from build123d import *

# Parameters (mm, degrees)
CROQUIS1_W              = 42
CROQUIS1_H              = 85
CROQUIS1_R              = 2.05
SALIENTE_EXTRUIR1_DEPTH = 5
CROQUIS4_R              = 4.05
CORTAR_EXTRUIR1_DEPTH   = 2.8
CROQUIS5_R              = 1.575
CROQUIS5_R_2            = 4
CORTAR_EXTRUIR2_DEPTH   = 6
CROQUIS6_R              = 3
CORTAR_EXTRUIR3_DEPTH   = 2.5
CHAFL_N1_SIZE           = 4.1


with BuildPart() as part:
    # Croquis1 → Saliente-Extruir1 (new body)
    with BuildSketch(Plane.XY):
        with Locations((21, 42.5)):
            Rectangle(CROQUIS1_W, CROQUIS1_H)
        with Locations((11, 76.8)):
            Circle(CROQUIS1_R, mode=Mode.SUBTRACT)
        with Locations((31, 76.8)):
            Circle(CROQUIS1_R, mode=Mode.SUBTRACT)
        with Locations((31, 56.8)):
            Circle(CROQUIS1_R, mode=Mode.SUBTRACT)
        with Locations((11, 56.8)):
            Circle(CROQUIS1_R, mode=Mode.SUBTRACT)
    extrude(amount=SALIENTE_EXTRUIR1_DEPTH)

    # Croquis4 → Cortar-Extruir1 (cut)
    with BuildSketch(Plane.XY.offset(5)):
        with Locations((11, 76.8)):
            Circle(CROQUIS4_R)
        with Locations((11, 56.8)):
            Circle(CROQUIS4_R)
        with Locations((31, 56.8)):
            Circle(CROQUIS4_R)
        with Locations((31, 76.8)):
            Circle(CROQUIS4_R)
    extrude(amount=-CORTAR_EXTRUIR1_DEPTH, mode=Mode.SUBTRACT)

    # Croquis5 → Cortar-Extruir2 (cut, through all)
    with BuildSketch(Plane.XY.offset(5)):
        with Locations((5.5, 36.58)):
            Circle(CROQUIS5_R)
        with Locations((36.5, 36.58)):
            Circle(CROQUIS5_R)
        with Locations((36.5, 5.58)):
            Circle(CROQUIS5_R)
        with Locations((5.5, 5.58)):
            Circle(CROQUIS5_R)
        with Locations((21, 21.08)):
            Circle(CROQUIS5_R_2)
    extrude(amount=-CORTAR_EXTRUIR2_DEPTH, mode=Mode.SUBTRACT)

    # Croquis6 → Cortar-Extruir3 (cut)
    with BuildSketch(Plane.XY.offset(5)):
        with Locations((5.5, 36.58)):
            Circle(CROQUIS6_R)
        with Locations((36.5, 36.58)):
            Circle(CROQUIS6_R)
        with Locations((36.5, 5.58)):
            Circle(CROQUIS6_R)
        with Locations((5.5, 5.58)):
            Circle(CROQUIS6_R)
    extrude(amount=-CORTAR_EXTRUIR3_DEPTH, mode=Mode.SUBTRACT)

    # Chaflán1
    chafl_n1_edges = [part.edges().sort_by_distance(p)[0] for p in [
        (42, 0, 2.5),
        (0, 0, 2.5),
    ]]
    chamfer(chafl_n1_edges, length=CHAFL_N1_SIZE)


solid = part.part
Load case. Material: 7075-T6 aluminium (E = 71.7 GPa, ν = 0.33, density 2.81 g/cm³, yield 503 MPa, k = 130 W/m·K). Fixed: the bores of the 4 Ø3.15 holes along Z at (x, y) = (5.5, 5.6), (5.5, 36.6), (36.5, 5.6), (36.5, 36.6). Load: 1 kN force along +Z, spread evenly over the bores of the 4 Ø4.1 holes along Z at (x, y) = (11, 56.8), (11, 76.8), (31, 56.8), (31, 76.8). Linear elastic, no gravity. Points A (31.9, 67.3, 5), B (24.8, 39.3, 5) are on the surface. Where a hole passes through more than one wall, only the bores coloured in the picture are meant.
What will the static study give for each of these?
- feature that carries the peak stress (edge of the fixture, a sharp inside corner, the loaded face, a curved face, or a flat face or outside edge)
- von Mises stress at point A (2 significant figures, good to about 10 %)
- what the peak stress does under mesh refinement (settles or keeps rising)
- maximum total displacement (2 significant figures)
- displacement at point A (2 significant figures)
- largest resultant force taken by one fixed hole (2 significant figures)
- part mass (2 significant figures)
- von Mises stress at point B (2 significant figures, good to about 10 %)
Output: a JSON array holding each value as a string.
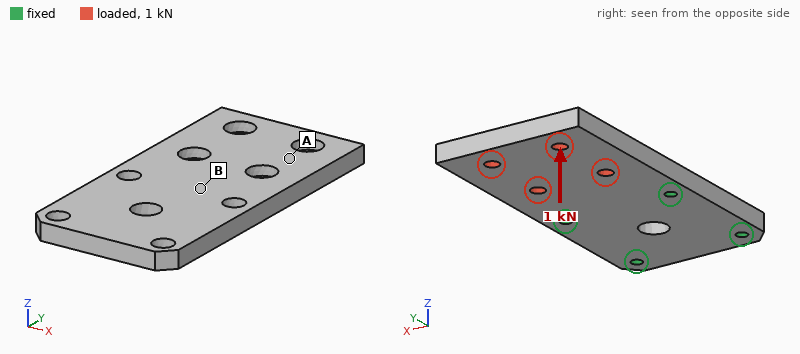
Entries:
["edge of the fixture", "33 MPa", "keeps rising", "0.91 mm", "0.50 mm", "1.4 kN", "46 g", "140 MPa"]
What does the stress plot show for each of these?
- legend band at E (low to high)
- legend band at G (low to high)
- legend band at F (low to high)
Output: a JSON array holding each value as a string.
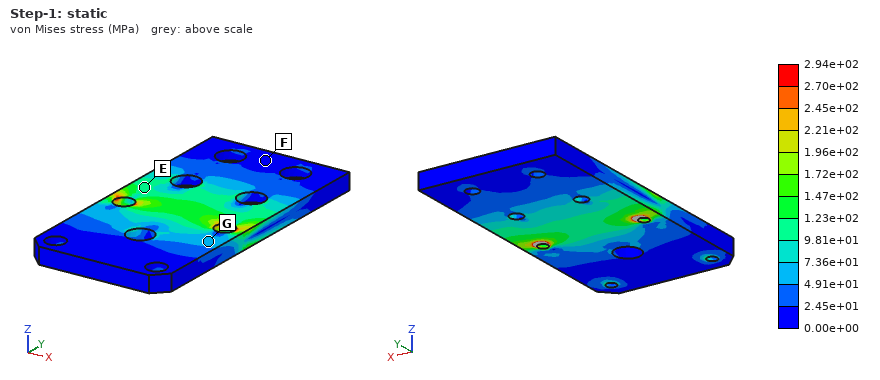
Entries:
["9.81e+01 to 1.23e+02 MPa", "4.91e+01 to 7.36e+01 MPa", "0.00e+00 to 2.45e+01 MPa"]
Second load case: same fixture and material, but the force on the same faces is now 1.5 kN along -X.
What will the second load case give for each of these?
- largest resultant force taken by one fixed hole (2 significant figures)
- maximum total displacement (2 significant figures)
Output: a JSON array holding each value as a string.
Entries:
["1.4 kN", "49 µm"]
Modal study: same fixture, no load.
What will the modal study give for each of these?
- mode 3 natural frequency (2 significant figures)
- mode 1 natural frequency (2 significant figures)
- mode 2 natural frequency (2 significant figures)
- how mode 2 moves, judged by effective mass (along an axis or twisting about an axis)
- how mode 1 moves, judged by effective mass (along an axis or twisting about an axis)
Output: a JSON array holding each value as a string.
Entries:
["8700 Hz", "1500 Hz", "4200 Hz", "twisting about Y", "along Z"]
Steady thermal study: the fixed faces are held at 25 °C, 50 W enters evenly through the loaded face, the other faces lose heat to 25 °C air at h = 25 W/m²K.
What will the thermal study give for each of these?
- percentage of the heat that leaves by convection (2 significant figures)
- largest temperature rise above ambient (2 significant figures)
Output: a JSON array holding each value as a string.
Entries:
["12 %", "71 K"]
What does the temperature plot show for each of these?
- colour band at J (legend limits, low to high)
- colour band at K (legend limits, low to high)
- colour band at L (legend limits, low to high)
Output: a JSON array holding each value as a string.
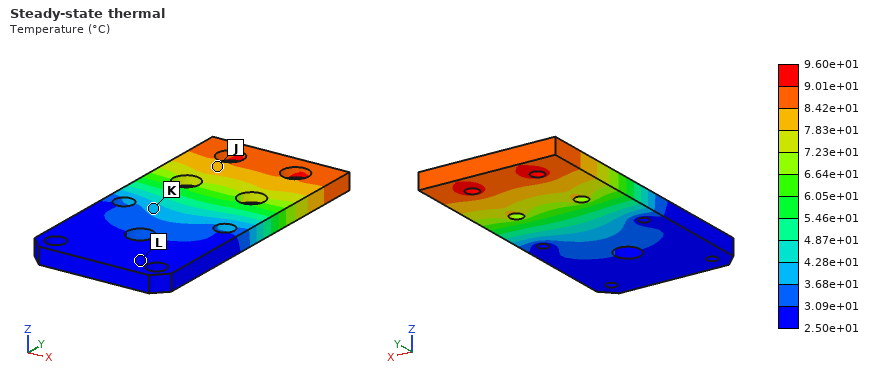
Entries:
["7.83e+01 to 8.42e+01 °C", "3.68e+01 to 4.28e+01 °C", "2.50e+01 to 3.09e+01 °C"]
